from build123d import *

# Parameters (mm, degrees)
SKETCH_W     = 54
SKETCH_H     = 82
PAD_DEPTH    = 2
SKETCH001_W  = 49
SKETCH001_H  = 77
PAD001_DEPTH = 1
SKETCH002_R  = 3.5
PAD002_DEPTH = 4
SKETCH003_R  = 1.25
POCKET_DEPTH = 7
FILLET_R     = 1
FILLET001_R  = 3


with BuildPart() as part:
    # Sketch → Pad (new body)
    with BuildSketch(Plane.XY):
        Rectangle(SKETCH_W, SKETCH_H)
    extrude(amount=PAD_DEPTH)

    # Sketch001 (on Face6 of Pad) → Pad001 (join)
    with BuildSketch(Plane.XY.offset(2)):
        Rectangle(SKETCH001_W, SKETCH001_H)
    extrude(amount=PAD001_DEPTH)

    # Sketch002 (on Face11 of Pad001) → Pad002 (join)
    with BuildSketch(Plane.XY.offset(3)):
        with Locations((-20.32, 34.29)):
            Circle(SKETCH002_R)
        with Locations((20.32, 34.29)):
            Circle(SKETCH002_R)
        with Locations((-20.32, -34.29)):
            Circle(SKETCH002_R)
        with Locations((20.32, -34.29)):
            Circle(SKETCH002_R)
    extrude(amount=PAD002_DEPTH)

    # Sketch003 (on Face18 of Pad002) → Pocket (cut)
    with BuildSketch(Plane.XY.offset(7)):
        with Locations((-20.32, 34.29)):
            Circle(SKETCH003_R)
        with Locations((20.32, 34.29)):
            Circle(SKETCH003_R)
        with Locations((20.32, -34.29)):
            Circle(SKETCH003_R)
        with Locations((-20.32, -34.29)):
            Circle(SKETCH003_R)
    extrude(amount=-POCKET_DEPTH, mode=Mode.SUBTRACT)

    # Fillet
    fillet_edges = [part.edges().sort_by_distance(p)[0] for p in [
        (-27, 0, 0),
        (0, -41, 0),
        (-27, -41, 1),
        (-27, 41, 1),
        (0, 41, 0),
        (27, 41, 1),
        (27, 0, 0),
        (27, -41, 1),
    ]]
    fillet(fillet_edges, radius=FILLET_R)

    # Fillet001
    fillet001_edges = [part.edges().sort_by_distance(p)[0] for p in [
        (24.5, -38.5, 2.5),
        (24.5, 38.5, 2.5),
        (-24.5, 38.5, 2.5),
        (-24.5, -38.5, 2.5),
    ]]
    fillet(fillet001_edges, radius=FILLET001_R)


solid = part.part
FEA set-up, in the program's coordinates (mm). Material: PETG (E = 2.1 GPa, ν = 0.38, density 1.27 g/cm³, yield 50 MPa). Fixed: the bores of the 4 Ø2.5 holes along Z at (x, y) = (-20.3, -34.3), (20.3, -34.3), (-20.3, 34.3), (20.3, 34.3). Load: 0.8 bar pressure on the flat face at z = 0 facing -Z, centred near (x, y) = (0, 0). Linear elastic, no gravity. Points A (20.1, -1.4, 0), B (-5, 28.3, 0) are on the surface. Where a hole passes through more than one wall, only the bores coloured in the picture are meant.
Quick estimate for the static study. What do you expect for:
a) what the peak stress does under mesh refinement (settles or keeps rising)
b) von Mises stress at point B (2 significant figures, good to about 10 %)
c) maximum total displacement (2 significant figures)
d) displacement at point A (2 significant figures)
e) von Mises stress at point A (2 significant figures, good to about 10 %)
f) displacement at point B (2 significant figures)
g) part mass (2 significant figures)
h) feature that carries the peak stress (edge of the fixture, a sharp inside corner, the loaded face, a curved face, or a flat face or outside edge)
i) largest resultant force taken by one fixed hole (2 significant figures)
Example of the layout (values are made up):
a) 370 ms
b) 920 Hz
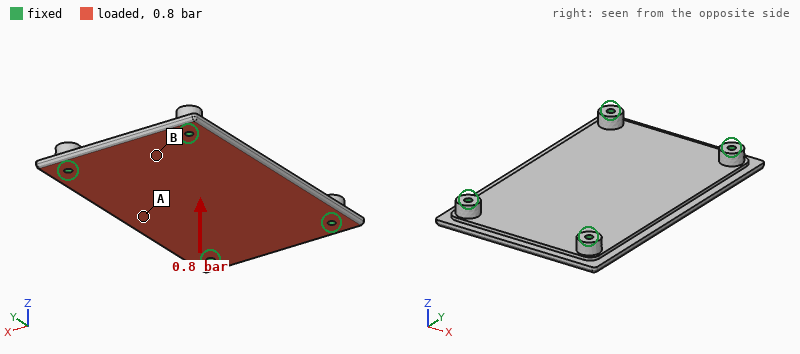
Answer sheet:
a) keeps rising
b) 5.7 MPa
c) 1.2 mm
d) 1.1 mm
e) 11 MPa
f) 0.32 mm
g) 17 g
h) edge of the fixture
i) 86 N
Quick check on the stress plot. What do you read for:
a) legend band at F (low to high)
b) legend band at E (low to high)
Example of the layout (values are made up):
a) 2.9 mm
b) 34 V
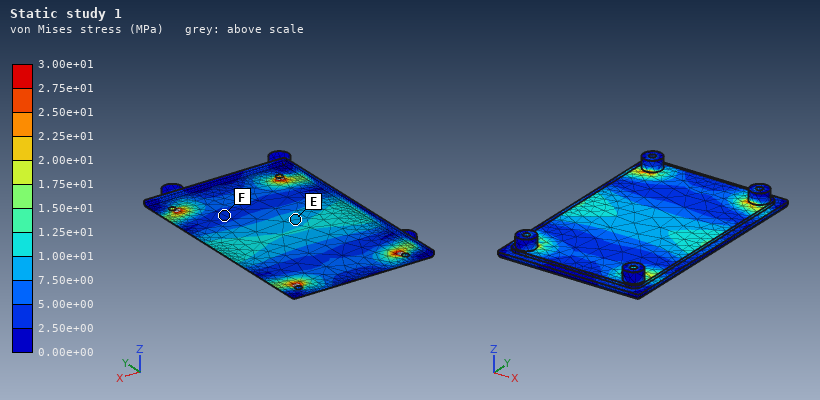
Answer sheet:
a) 2.50e+00 to 5.00e+00 MPa
b) 7.50e+00 to 1.00e+01 MPa
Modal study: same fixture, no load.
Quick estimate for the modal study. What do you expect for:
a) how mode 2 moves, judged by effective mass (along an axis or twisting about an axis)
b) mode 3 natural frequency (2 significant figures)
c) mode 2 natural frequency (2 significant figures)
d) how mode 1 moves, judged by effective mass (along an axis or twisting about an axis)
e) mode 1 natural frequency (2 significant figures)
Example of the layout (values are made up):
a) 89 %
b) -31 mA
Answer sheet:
a) twisting about Y
b) 2000 Hz
c) 1100 Hz
d) along Z
e) 780 Hz
